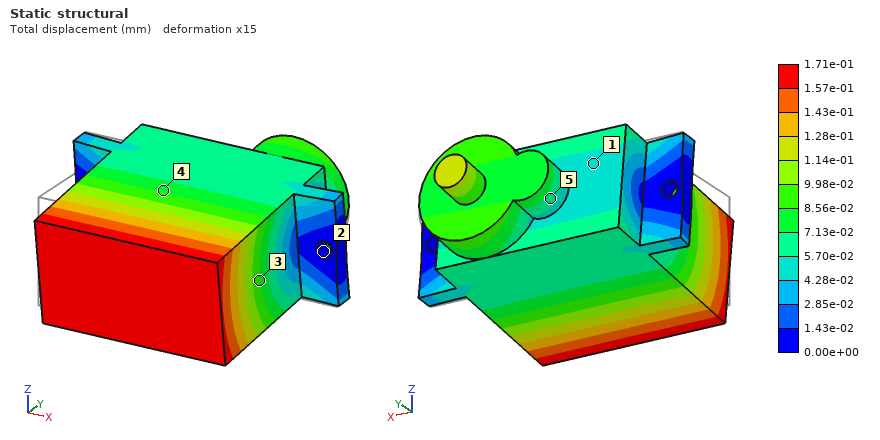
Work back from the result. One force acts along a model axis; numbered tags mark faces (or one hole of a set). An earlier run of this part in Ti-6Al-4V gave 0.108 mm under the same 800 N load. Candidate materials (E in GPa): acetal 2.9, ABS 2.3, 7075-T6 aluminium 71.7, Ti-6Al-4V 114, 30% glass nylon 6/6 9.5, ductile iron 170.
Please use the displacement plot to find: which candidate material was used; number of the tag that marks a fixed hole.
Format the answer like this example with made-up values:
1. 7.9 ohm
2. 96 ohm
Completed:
1. 7075-T6 aluminium
2. 2
